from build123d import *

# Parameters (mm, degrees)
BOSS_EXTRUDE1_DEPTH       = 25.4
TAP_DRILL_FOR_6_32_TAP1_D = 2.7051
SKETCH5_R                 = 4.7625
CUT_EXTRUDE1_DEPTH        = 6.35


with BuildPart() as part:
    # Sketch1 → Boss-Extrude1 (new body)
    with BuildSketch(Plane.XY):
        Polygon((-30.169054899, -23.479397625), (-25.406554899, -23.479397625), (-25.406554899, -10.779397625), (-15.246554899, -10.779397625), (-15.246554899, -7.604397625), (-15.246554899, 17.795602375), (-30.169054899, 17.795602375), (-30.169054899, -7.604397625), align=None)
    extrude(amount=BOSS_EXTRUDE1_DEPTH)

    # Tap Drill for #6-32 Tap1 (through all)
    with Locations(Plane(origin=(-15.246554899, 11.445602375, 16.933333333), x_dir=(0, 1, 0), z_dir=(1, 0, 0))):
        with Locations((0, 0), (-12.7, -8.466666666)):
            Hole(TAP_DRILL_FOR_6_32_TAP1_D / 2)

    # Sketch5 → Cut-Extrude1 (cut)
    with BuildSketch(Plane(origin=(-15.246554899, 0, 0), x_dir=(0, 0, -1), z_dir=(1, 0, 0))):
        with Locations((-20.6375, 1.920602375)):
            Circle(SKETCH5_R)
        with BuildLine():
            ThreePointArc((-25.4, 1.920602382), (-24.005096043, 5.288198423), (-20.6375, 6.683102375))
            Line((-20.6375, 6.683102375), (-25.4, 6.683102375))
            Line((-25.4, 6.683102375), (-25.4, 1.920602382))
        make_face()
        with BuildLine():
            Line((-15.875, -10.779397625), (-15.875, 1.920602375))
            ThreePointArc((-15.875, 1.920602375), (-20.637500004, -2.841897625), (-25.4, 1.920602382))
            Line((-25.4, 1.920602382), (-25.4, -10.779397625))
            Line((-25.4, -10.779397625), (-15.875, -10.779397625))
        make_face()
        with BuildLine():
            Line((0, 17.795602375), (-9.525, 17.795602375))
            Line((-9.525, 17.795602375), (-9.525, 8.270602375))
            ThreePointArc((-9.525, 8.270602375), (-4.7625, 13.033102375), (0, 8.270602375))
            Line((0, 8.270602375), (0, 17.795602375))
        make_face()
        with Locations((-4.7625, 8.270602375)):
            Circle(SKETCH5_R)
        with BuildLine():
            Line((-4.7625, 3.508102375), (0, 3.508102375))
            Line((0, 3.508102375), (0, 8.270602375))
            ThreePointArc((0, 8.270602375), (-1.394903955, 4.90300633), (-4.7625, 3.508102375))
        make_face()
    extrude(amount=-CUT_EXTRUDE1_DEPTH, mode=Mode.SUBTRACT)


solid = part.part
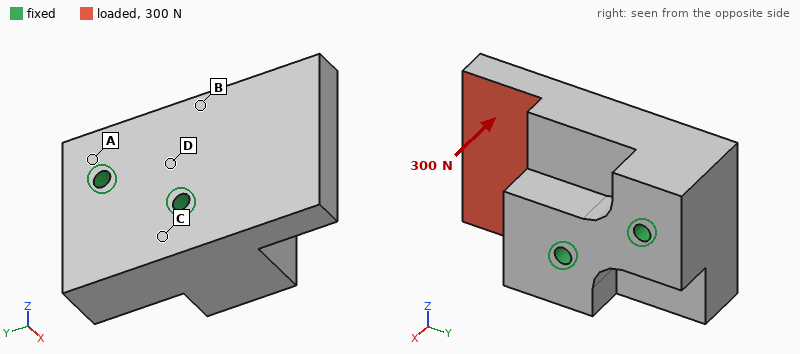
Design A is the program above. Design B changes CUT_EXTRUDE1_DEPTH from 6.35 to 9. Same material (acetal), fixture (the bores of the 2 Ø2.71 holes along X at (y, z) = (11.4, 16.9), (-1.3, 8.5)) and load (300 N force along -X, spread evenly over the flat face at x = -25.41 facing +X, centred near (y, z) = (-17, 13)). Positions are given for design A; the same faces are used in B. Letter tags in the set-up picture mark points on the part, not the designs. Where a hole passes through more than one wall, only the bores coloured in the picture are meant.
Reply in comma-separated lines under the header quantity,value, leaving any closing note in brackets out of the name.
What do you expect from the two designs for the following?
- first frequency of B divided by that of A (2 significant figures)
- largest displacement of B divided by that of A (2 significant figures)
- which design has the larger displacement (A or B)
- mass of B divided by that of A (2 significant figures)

quantity,value
first frequency of B divided by that of A,0.94
largest displacement of B divided by that of A,1.2
which design has the larger displacement,B
mass of B divided by that of A,0.92
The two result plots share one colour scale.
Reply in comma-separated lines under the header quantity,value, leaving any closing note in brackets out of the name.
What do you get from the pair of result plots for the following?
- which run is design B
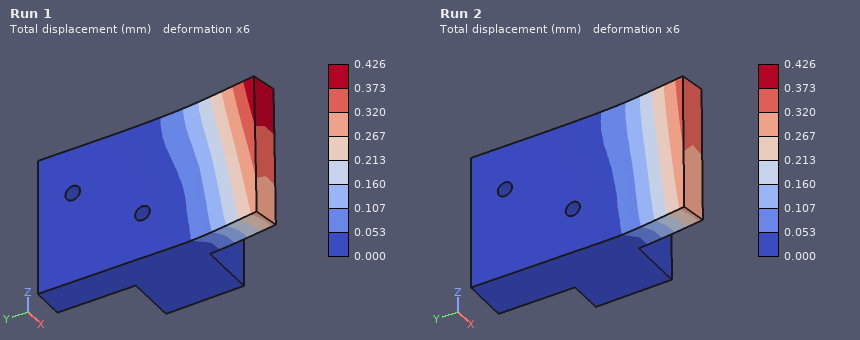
quantity,value
which run is design B,Run 1
